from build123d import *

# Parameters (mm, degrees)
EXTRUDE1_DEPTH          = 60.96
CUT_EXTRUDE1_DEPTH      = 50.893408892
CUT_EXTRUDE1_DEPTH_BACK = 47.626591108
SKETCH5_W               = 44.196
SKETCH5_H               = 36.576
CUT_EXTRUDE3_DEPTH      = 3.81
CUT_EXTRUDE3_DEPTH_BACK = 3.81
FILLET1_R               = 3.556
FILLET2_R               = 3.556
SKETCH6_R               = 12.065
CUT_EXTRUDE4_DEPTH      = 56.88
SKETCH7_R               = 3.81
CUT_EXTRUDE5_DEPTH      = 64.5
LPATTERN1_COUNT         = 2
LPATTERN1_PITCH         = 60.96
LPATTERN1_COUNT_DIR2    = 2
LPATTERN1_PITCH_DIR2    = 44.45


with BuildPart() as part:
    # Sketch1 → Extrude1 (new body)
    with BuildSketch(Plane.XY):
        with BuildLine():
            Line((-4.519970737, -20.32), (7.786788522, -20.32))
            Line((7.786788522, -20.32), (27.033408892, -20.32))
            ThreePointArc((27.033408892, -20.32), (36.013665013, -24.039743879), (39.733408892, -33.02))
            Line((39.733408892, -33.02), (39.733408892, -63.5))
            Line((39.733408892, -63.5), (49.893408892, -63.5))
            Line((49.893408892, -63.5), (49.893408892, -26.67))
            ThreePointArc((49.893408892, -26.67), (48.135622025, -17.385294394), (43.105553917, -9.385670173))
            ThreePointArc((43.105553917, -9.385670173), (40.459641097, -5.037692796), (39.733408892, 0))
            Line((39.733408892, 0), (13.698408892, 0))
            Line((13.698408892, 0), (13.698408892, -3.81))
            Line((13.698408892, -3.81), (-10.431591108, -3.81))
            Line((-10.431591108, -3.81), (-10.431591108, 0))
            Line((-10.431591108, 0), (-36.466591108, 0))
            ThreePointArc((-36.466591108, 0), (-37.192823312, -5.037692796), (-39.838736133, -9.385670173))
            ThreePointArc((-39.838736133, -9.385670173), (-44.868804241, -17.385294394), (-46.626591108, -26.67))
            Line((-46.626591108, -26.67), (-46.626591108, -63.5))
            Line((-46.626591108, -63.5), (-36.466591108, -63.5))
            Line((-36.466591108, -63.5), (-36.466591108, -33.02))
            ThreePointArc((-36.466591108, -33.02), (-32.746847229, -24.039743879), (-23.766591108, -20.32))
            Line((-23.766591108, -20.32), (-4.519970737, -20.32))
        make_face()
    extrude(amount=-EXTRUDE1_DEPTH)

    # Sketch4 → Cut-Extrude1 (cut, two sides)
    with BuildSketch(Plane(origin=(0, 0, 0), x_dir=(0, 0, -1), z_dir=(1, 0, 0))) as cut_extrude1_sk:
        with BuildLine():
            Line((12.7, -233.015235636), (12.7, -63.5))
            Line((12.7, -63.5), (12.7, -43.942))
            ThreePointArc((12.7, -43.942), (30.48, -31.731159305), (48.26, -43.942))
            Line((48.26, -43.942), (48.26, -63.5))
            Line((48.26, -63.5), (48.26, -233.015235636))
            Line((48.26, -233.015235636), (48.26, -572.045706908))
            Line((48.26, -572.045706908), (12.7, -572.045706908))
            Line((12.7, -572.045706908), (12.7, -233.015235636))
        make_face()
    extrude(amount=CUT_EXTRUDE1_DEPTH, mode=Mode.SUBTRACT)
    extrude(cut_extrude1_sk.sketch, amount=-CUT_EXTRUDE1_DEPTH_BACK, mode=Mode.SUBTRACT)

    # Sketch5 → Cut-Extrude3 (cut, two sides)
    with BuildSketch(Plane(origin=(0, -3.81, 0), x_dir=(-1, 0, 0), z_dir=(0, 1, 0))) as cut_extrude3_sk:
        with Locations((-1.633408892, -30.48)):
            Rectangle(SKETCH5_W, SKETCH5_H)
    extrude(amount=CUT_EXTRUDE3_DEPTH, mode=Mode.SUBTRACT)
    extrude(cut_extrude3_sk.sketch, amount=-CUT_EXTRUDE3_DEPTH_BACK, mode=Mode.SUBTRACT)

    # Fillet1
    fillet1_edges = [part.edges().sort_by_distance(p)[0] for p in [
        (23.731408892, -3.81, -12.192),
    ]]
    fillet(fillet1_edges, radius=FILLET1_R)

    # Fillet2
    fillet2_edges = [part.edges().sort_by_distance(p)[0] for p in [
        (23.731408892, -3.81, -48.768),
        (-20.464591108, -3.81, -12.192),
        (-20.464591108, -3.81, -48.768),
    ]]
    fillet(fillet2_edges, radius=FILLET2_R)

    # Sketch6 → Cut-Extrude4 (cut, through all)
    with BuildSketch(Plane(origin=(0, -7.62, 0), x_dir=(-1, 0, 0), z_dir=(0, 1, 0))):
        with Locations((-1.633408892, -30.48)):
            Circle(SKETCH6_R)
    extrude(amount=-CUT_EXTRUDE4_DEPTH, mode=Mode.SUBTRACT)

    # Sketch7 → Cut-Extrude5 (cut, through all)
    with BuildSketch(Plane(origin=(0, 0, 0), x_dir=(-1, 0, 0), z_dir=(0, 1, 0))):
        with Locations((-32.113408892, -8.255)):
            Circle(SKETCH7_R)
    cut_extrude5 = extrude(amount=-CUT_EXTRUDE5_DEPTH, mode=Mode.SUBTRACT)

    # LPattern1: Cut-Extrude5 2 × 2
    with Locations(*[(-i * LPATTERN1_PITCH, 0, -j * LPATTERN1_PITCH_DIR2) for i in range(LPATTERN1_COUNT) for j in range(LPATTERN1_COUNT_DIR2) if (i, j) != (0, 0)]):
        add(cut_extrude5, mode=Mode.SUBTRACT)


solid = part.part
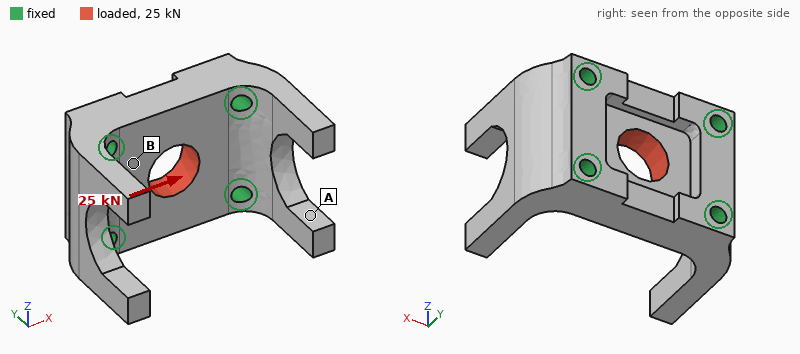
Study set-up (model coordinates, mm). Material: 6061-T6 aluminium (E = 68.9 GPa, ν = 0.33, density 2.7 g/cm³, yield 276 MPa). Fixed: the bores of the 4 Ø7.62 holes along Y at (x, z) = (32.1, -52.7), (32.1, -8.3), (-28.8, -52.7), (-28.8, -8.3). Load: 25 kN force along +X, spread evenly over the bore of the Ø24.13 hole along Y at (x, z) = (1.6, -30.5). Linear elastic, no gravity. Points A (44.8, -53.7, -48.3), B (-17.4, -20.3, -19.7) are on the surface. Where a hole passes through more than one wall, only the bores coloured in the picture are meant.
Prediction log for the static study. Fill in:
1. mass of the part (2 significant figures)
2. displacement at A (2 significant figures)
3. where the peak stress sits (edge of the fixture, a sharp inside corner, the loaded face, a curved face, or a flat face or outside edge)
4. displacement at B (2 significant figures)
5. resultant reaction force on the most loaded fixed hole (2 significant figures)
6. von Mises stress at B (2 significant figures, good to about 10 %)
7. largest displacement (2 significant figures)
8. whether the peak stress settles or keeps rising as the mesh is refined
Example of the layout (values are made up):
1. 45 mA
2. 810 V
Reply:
1. 320 g
2. 3.1 µm
3. edge of the fixture
4. 5.5 µm
5. 6.5 kN
6. 22 MPa
7. 10 µm
8. keeps rising
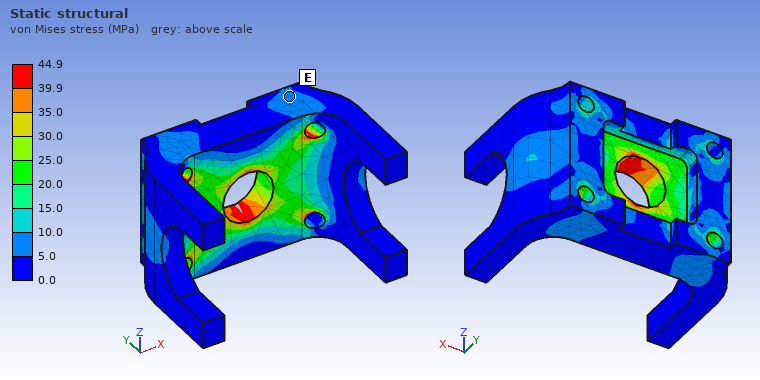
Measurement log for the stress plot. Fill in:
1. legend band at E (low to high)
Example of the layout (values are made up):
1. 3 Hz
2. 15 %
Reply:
1. 5.0 to 10.0 MPa
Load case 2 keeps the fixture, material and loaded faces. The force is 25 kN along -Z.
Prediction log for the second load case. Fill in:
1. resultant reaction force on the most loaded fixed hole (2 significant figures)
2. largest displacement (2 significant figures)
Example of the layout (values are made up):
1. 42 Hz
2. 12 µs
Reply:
1. 7.2 kN
2. 20 µm
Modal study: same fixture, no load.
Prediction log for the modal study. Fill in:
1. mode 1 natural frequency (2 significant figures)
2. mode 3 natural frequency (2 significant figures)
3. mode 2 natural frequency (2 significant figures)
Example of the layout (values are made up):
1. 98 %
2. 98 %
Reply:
1. 5300 Hz
2. 5400 Hz
3. 5300 Hz
